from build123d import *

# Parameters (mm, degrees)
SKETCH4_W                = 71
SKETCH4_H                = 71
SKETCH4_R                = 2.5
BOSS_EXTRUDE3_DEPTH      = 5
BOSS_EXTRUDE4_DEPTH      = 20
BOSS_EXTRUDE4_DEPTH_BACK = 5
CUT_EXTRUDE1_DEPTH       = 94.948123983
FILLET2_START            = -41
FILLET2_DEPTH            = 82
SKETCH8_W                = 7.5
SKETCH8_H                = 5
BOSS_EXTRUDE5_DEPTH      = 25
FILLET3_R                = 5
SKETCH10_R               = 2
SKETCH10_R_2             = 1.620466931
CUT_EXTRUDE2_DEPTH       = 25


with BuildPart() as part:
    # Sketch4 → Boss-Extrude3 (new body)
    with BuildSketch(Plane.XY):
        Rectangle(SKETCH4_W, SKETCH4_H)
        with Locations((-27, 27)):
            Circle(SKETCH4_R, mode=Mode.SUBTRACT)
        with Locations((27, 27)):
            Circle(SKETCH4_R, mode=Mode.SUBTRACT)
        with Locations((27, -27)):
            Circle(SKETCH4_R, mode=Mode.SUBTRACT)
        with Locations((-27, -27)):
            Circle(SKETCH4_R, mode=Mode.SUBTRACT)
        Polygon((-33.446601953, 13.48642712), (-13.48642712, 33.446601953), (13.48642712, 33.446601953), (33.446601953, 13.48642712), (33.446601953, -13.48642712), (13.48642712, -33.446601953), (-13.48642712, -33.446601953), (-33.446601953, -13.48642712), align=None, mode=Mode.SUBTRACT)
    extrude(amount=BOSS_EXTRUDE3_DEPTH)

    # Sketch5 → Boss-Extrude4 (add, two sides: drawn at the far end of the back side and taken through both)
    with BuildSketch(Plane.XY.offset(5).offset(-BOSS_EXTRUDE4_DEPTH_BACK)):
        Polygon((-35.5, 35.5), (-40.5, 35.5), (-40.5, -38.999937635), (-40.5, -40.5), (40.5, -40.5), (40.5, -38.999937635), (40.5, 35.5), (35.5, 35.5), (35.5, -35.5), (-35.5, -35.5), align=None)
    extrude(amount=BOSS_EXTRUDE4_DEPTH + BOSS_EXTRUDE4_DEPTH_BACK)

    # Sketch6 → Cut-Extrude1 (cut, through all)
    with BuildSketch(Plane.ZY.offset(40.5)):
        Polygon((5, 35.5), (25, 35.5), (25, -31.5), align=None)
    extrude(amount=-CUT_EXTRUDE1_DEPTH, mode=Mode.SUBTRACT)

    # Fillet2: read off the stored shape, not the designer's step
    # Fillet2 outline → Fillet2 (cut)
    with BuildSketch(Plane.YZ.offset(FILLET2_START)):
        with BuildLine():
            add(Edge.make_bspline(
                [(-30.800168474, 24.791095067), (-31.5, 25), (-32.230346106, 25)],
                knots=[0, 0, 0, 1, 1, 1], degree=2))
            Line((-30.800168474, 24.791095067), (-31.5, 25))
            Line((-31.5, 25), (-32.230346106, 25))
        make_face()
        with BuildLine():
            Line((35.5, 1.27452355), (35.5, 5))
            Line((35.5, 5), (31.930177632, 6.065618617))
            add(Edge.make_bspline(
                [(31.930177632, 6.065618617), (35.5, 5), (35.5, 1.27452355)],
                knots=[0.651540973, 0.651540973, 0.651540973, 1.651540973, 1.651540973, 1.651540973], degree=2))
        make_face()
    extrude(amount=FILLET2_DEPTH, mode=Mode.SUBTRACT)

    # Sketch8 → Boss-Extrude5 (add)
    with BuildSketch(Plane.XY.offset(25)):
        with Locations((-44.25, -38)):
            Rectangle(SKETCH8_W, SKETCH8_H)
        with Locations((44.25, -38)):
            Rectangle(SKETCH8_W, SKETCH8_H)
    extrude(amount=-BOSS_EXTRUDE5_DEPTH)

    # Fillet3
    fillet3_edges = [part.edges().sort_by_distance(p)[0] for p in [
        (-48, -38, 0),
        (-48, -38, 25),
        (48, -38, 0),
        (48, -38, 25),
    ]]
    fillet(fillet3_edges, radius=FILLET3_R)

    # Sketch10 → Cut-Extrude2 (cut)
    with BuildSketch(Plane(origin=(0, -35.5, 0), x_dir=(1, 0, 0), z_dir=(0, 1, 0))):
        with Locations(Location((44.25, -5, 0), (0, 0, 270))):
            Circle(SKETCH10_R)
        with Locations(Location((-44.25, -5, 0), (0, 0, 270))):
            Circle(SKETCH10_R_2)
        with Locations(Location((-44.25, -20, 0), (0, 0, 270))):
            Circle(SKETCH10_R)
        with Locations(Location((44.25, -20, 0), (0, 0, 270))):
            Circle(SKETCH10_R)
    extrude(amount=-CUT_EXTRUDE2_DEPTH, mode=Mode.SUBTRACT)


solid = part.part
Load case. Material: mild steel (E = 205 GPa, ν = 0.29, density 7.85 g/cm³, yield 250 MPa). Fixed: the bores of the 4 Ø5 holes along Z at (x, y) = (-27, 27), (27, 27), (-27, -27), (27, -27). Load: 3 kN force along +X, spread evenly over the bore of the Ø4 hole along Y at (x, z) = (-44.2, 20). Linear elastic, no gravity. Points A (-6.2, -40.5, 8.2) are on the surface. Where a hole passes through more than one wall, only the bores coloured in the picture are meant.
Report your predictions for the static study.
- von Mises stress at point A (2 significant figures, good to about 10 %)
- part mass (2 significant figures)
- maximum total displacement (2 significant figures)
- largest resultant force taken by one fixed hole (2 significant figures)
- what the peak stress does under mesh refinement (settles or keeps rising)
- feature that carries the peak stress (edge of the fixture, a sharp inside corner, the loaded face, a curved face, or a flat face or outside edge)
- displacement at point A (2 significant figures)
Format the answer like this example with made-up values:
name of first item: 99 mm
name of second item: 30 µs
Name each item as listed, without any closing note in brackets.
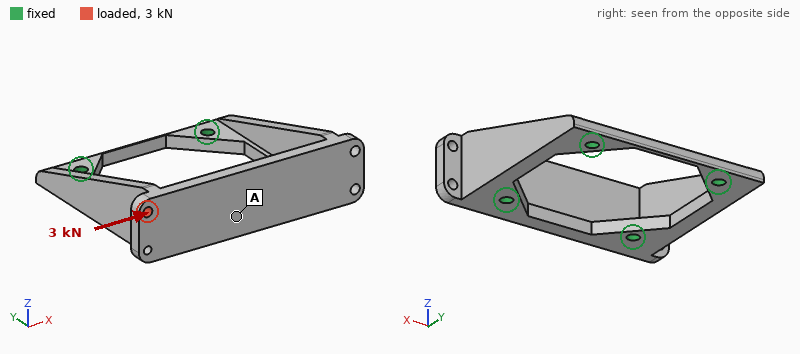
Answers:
von Mises stress at point A: 21 MPa
part mass: 230 g
maximum total displacement: 26 µm
largest resultant force taken by one fixed hole: 1.8 kN
what the peak stress does under mesh refinement: keeps rising
feature that carries the peak stress: edge of the fixture
displacement at point A: 5.5 µm
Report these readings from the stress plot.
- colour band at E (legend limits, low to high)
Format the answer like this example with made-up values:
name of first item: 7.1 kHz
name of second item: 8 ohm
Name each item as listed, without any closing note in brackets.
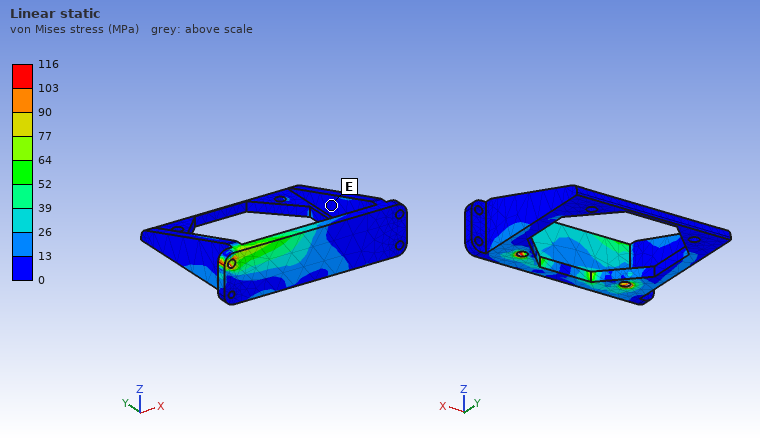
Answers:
colour band at E: 0 to 13 MPa
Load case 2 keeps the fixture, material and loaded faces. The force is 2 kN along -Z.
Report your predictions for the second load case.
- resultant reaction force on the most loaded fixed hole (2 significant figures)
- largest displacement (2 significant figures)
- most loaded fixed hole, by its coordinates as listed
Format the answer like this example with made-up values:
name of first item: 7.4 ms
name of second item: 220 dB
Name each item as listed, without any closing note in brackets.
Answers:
resultant reaction force on the most loaded fixed hole: 2.8 kN
largest displacement: 32 µm
most loaded fixed hole, by its coordinates as listed: (-27, -27)
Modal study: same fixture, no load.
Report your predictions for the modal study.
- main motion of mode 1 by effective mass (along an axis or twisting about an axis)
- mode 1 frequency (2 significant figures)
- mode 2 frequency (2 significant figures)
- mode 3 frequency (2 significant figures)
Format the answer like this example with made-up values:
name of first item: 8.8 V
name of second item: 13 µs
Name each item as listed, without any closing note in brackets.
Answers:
main motion of mode 1 by effective mass: along Y
mode 1 frequency: 5600 Hz
mode 2 frequency: 7500 Hz
mode 3 frequency: 7800 Hz
